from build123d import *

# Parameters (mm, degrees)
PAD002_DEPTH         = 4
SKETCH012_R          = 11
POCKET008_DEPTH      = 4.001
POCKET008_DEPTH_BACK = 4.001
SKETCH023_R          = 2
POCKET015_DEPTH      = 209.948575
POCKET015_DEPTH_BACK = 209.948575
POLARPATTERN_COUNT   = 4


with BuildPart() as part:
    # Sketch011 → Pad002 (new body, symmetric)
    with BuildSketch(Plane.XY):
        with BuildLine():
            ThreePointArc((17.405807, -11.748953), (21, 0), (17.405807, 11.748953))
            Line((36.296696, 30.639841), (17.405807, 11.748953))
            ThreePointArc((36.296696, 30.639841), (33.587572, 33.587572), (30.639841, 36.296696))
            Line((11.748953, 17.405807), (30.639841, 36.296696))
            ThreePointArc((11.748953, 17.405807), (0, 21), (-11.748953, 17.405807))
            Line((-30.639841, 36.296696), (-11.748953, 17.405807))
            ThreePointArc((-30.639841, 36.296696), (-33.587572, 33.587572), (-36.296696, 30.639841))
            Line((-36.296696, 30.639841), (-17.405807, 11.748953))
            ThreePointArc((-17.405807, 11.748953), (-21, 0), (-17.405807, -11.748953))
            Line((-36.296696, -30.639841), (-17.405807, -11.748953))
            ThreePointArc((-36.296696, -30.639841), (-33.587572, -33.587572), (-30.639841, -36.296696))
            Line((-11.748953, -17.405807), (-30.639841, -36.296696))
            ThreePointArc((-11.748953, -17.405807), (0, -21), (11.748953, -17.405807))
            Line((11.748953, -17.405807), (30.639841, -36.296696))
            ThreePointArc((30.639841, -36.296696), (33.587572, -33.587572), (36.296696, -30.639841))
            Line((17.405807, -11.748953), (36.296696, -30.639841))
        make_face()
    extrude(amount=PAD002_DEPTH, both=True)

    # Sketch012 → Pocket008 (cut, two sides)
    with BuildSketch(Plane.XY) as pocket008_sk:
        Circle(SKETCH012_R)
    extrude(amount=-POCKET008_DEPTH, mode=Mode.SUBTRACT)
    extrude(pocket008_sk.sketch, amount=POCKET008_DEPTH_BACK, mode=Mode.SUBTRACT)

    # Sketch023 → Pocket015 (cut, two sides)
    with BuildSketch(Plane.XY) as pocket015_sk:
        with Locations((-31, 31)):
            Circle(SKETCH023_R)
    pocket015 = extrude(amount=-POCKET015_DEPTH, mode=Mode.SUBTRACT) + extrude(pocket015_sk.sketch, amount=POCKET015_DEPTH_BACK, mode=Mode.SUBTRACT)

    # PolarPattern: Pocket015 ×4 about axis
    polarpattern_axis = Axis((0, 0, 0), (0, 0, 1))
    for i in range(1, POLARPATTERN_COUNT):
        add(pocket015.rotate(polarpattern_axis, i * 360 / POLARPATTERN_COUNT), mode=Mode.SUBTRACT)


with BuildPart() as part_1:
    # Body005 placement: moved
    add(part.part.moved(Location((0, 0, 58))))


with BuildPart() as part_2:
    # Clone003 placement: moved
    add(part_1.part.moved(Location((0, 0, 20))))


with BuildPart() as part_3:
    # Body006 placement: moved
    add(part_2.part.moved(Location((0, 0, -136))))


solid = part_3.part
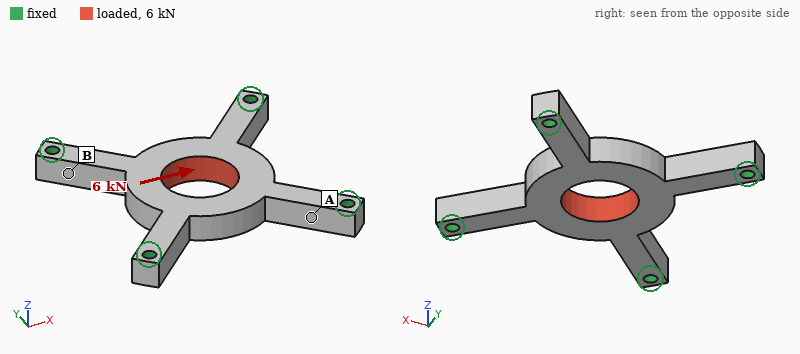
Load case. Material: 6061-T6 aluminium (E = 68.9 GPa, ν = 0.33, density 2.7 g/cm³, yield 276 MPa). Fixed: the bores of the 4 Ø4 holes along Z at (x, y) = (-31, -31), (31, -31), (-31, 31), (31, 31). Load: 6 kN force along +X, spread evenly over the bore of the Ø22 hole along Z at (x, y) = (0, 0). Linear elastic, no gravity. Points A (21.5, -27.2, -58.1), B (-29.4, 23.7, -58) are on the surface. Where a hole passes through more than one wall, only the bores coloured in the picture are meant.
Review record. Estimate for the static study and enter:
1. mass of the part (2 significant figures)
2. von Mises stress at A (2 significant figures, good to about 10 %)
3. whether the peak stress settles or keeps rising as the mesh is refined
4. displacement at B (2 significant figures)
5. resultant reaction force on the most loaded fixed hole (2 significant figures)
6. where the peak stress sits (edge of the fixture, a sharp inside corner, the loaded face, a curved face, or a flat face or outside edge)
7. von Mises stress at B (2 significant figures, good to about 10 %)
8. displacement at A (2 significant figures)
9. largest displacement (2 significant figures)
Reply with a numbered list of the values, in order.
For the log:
1. 39 g
2. 23 MPa
3. keeps rising
4. 5.2 µm
5. 2.0 kN
6. edge of the fixture
7. 42 MPa
8. 3.8 µm
9. 25 µm
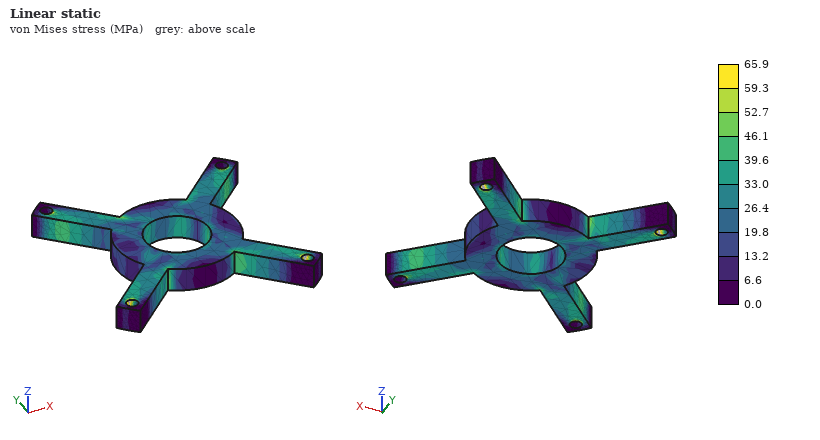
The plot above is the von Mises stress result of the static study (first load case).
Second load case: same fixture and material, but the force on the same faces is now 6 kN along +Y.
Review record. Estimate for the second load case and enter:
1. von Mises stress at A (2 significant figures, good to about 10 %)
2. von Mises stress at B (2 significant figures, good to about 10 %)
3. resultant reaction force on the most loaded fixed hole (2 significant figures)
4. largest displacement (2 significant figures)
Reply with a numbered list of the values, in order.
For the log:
1. 40 MPa
2. 15 MPa
3. 2.0 kN
4. 25 µm
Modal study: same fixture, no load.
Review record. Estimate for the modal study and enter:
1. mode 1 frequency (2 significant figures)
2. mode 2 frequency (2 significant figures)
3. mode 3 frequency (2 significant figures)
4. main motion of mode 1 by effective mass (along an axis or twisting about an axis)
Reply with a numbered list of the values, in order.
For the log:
1. 5700 Hz
2. 10 kHz
3. 10 kHz
4. along Z
